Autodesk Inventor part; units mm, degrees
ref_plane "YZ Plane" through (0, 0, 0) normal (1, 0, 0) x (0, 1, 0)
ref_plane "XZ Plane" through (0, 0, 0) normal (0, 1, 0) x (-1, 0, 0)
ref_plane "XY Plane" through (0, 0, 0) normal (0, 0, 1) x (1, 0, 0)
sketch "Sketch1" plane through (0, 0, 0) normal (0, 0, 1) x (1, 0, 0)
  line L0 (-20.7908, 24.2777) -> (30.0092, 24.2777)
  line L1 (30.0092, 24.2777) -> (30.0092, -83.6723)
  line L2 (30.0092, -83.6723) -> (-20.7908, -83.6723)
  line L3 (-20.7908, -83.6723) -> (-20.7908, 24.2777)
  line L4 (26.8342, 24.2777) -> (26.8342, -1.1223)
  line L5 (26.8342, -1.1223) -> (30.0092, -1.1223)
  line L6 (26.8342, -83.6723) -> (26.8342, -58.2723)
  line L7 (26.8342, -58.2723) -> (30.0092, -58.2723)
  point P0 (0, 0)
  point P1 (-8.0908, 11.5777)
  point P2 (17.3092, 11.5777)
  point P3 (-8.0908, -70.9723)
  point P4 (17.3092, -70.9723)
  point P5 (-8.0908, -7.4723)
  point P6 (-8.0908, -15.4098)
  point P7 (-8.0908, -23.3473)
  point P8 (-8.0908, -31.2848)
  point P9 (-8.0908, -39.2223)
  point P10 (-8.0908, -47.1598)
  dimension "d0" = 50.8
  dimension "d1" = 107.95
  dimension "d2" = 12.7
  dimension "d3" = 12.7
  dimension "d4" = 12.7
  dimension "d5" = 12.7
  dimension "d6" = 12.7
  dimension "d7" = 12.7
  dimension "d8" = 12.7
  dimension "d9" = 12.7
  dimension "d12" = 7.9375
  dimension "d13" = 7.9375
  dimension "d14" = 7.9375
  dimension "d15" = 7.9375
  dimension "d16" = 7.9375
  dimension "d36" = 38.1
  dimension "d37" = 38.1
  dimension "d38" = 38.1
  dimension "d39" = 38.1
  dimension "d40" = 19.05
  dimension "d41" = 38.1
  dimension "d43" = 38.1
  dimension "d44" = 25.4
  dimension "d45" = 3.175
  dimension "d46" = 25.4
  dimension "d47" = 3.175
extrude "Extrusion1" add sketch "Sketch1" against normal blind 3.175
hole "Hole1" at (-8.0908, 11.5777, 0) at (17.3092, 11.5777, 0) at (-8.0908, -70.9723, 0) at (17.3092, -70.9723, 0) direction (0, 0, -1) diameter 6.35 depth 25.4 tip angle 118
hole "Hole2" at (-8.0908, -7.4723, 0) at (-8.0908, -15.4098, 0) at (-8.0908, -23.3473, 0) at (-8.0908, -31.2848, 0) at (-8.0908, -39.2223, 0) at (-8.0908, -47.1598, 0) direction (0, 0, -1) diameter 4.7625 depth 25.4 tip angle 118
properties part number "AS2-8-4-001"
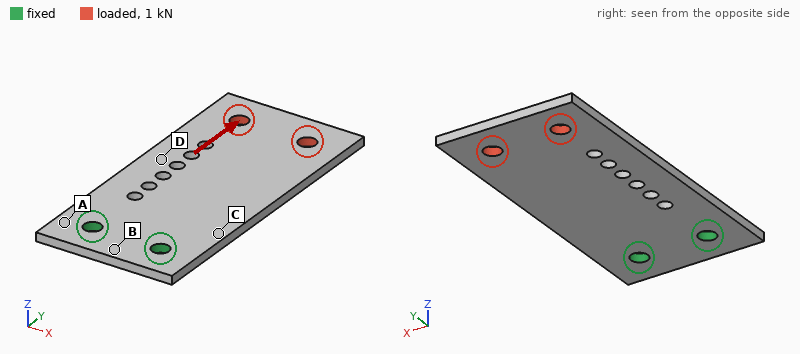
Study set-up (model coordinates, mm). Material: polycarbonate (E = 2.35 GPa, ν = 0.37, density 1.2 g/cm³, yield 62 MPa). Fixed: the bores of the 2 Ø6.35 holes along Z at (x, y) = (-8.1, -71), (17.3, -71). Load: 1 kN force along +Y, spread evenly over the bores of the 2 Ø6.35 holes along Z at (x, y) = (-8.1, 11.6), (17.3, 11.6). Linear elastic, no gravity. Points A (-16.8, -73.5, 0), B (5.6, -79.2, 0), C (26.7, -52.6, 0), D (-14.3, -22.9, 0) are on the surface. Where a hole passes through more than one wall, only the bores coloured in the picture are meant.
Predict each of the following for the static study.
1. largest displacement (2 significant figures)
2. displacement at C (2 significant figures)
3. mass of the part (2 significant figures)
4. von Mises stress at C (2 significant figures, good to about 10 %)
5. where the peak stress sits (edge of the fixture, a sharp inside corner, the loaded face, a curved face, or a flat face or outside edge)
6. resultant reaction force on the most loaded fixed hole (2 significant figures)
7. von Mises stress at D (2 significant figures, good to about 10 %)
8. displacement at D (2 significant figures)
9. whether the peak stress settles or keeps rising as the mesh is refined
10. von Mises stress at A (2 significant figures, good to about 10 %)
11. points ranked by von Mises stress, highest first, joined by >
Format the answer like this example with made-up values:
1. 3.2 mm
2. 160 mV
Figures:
1. 0.28 mm
2. 0.065 mm
3. 20 g
4. 5.4 MPa
5. edge of the fixture
6. 500 N
7. 6.9 MPa
8. 0.15 mm
9. keeps rising
10. 2.8 MPa
11. D > C > A > B
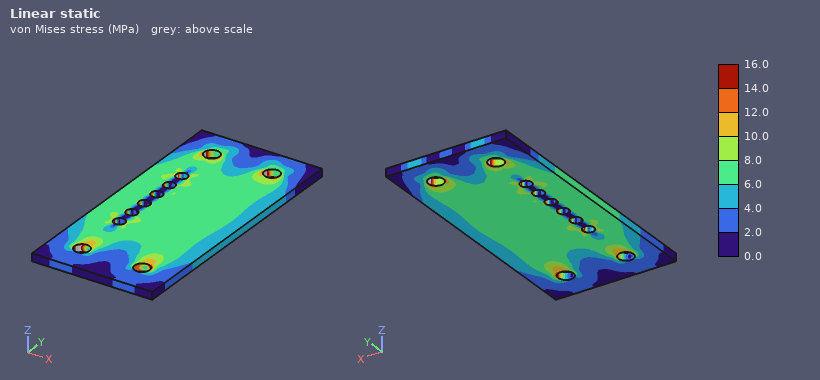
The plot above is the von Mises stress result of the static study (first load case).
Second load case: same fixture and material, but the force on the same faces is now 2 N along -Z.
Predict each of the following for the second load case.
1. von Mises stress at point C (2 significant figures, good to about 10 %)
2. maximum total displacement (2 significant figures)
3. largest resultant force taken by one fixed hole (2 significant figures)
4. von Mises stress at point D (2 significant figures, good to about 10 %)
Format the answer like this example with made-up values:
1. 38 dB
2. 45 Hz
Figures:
1. 1.6 MPa
2. 1.4 mm
3. 1.0 N
4. 0.89 MPa
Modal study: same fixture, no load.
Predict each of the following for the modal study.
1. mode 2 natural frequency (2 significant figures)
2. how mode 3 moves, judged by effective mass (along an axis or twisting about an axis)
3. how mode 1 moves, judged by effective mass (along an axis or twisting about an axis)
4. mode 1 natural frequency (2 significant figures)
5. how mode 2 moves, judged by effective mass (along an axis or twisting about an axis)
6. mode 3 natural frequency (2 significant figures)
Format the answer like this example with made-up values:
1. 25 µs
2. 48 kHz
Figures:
1. 310 Hz
2. along Z
3. along Z
4. 84 Hz
5. twisting about Y
6. 510 Hz
